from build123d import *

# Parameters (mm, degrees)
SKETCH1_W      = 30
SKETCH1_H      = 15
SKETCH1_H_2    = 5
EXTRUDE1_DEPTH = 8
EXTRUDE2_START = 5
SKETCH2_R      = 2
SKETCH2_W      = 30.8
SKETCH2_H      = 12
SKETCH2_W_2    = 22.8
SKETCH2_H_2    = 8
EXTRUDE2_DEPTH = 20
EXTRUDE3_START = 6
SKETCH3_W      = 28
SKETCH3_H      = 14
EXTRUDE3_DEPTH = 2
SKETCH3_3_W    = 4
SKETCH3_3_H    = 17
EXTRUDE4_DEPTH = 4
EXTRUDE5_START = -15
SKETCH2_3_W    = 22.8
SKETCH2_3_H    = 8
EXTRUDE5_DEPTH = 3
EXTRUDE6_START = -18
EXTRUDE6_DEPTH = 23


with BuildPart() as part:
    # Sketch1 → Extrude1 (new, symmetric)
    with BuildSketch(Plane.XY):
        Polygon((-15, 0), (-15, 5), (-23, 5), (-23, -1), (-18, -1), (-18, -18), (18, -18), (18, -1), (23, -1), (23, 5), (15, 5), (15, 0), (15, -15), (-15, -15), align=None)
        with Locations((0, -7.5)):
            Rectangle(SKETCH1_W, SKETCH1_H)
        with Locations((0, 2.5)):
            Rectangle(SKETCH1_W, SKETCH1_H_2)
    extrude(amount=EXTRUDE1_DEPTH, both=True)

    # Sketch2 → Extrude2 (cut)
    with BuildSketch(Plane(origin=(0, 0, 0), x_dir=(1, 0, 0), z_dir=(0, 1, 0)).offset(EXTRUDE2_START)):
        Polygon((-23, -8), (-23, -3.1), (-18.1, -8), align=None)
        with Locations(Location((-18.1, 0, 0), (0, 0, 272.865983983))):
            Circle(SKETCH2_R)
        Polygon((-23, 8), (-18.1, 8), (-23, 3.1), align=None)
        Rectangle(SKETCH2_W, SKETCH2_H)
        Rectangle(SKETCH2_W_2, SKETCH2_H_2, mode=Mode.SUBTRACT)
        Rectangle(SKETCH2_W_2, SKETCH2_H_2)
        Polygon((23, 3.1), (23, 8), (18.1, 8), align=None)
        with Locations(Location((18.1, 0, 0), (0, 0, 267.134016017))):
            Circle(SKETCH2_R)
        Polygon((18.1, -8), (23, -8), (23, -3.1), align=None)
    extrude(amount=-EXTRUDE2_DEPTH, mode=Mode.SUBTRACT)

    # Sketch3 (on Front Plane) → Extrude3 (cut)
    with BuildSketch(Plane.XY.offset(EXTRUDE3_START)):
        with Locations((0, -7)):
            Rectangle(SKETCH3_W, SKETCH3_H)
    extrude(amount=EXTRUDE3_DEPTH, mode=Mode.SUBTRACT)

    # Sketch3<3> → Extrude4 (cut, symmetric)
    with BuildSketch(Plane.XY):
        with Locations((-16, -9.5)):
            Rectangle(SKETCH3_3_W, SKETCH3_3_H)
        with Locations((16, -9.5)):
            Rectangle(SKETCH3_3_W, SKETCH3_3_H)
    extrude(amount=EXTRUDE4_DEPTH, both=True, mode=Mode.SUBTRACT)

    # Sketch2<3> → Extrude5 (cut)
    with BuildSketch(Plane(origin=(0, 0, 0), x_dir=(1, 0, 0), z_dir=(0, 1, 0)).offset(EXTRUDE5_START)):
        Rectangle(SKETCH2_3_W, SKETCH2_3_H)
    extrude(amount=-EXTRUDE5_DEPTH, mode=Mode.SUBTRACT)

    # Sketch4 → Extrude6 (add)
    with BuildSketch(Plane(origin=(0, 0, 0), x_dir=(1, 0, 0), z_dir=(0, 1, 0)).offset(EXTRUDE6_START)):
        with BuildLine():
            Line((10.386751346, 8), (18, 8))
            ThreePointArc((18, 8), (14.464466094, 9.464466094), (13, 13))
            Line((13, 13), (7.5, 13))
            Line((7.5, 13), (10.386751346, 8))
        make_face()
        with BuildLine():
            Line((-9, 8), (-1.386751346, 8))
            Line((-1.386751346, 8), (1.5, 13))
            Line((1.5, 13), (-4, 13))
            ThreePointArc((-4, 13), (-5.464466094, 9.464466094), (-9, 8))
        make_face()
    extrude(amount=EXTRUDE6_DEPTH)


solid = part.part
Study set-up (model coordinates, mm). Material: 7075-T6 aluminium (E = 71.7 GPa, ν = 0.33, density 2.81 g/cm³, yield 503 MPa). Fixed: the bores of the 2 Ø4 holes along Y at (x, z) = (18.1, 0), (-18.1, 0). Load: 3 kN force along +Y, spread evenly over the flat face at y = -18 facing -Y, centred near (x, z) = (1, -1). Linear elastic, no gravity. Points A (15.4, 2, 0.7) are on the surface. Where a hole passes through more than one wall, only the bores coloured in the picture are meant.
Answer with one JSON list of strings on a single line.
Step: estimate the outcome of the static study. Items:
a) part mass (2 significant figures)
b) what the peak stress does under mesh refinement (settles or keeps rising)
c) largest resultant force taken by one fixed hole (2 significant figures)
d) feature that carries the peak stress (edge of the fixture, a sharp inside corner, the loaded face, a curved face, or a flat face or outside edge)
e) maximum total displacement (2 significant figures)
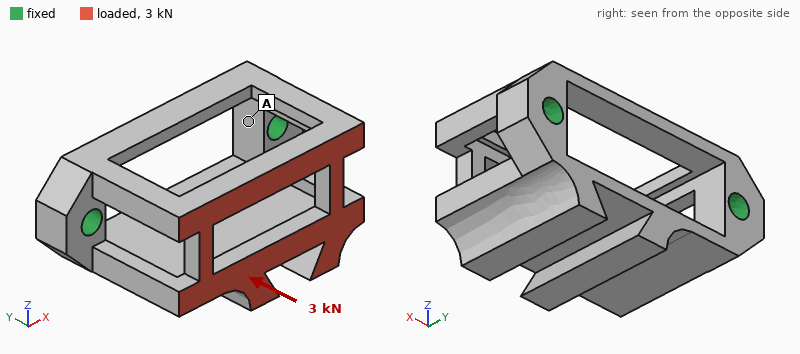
["15 g", "keeps rising", "1.6 kN", "a sharp inside corner", "0.16 mm"]
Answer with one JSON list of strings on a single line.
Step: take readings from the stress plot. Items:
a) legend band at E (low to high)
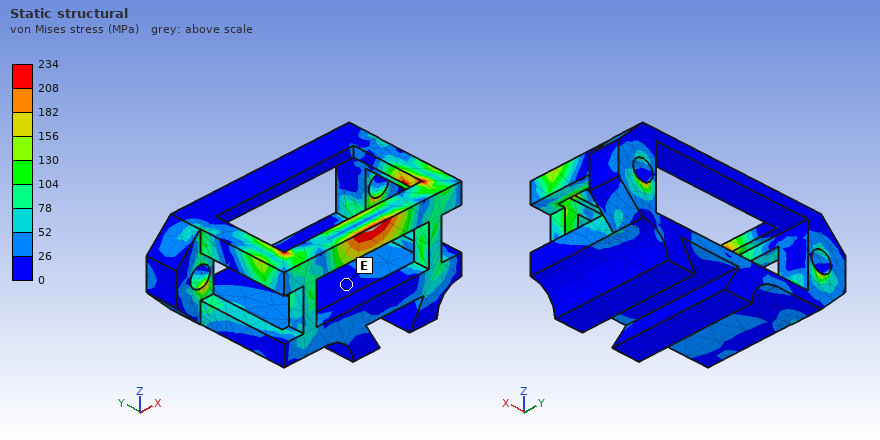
["0 to 26 MPa"]
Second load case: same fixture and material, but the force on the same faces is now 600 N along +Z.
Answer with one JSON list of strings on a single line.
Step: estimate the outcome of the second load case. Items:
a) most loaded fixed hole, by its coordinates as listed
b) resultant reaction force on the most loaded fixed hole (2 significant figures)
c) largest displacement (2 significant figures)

["(18.1, 0)", "320 N", "0.16 mm"]
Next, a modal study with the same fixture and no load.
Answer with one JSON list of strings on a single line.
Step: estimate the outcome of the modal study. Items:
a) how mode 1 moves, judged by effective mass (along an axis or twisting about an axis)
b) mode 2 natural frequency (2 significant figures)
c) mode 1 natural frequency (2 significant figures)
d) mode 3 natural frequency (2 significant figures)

["along Z", "7900 Hz", "4700 Hz", "8500 Hz"]
